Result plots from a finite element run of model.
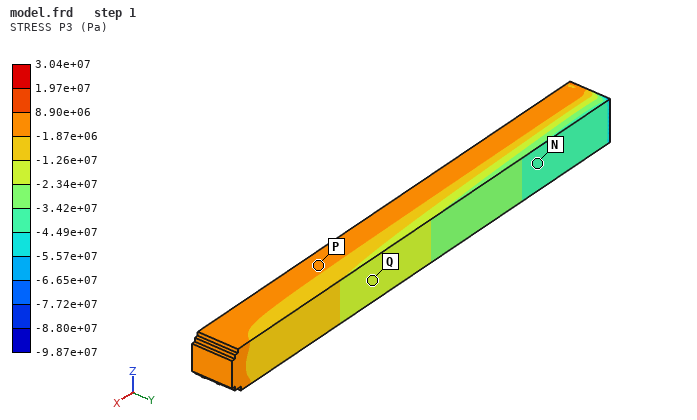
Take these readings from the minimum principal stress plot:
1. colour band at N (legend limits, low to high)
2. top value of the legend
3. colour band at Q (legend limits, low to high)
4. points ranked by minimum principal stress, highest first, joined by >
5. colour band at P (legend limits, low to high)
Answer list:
-4.49e+07 to -3.42e+07 Pa
3.04e+07 Pa
-2.34e+07 to -1.26e+07 Pa
P > Q > N
-1.87e+06 to 8.90e+06 Pa
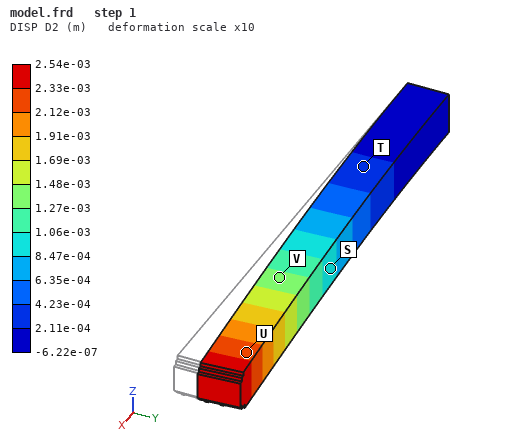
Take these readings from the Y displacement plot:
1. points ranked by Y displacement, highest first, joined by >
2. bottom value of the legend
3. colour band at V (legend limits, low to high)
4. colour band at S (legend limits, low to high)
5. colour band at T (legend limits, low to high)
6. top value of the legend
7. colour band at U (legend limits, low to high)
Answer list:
U > V > S > T
-6.22e-07 m
1.27e-03 to 1.48e-03 m
8.47e-04 to 1.06e-03 m
2.11e-04 to 4.23e-04 m
2.54e-03 m
2.12e-03 to 2.33e-03 m
